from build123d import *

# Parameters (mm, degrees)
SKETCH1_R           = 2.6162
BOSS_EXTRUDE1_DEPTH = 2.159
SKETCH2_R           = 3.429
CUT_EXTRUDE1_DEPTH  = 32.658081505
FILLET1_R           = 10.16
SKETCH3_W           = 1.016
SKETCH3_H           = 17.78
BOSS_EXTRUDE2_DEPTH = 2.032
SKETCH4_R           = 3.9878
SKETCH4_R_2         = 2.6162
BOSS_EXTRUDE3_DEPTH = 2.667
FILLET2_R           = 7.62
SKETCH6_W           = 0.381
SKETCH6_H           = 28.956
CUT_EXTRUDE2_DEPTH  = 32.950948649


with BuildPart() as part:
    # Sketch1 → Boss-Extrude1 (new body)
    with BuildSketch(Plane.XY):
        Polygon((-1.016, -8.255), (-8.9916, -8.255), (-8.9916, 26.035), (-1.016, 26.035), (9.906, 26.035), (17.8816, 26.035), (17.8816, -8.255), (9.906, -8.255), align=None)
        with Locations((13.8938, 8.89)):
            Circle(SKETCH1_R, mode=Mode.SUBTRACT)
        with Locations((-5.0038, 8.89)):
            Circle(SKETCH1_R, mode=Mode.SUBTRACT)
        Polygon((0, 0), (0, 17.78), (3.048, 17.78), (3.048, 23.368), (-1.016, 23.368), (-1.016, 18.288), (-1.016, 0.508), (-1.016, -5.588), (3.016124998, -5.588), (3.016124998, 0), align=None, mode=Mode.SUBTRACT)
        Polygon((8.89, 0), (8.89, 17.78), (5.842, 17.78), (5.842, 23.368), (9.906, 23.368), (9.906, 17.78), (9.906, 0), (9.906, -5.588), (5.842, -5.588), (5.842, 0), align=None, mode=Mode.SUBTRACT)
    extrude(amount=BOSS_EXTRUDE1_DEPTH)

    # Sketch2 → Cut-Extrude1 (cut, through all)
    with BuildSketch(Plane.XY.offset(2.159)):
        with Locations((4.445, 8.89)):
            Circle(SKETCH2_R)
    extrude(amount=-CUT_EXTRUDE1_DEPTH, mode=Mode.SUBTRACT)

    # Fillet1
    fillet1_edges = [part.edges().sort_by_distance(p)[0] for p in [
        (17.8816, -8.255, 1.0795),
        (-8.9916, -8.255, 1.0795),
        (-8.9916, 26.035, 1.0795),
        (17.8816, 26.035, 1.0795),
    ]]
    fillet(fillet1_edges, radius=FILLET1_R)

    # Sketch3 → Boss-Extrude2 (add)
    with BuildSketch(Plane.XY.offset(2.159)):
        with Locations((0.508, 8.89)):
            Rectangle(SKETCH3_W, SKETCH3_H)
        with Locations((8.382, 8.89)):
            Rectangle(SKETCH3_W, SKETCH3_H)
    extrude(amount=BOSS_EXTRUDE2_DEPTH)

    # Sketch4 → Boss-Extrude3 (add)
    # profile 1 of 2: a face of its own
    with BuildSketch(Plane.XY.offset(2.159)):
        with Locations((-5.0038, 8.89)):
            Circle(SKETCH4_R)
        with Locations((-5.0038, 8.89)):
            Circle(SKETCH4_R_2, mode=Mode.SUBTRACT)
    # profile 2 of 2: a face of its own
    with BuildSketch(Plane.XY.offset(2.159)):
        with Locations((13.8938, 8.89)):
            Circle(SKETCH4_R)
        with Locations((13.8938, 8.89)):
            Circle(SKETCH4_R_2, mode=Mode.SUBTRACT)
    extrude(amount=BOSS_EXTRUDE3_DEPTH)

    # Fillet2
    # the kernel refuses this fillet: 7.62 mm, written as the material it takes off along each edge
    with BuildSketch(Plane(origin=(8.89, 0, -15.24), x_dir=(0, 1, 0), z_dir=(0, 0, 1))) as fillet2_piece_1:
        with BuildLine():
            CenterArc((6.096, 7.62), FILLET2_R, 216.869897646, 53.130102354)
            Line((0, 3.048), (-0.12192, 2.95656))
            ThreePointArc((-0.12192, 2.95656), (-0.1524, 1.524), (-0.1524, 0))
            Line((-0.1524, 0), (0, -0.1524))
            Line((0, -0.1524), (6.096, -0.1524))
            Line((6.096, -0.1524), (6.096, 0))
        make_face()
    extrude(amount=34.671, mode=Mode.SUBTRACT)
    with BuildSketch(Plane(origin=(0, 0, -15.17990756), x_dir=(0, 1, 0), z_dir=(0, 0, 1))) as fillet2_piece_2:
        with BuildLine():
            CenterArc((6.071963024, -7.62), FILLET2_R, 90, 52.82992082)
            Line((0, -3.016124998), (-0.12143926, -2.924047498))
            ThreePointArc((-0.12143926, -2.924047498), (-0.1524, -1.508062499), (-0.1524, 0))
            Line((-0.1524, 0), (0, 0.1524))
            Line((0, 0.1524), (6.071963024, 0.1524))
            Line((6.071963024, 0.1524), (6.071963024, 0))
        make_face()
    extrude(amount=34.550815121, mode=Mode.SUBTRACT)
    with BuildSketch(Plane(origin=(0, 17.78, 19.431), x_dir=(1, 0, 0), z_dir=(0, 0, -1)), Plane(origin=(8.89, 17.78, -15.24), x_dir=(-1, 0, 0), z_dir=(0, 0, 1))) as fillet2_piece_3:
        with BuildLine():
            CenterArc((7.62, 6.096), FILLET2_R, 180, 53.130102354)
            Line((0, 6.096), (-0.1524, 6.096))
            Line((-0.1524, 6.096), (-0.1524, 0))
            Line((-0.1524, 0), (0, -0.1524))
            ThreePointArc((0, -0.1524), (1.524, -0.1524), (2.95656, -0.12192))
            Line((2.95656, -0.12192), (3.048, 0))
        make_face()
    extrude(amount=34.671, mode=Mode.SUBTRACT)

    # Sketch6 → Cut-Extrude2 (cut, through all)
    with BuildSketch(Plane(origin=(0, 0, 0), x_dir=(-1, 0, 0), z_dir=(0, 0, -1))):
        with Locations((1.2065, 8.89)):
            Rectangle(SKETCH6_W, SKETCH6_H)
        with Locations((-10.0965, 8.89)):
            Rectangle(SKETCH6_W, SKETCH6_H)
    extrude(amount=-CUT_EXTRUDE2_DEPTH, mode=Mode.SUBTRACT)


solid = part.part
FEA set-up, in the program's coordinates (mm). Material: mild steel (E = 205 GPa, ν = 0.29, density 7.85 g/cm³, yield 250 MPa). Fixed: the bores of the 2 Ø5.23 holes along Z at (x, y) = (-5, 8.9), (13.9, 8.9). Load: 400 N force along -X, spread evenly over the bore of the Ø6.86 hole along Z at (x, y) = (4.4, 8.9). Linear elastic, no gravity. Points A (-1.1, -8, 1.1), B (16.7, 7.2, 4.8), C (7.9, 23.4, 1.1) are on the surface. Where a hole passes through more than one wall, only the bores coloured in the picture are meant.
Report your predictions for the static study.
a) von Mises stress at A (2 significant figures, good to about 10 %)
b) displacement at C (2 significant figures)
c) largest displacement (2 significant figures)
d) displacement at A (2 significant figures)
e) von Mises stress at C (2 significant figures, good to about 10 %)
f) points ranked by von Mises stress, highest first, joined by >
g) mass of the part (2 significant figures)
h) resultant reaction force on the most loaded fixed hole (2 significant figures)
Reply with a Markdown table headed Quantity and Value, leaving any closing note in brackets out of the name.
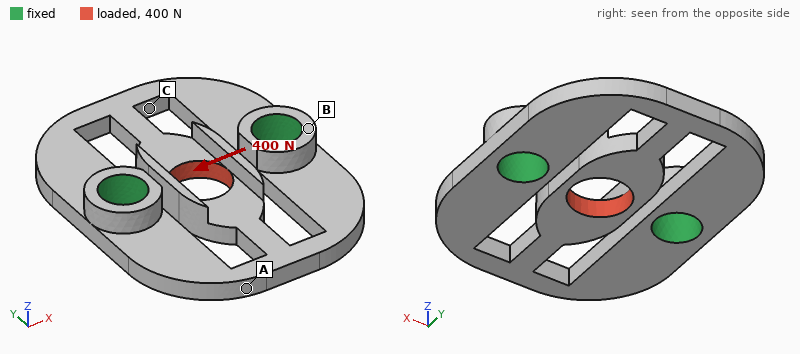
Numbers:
| Quantity | Value |
|---|---|
| von Mises stress at A | 51 MPa |
| displacement at C | 8.9 µm |
| largest displacement | 30 µm |
| displacement at A | 8.7 µm |
| von Mises stress at C | 110 MPa |
| points ranked by von Mises stress, highest first, joined by > | C > A > B |
| mass of the part | 11 g |
| resultant reaction force on the most loaded fixed hole | 200 N |
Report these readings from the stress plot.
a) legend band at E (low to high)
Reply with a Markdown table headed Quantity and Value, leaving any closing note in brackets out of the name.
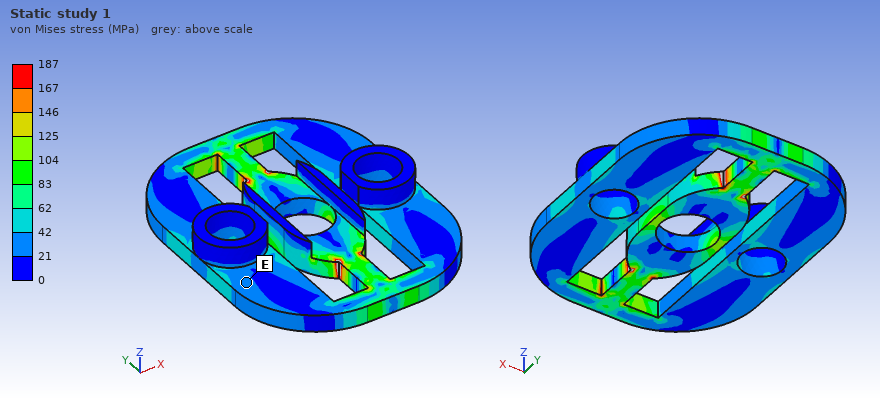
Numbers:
| Quantity | Value |
|---|---|
| legend band at E | 21 to 42 MPa |
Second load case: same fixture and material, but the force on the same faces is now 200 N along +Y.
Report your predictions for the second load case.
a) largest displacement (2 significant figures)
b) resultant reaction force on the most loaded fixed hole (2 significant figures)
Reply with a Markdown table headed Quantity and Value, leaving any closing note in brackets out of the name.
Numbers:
| Quantity | Value |
|---|---|
| largest displacement | 4.3 µm |
| resultant reaction force on the most loaded fixed hole | 100 N |
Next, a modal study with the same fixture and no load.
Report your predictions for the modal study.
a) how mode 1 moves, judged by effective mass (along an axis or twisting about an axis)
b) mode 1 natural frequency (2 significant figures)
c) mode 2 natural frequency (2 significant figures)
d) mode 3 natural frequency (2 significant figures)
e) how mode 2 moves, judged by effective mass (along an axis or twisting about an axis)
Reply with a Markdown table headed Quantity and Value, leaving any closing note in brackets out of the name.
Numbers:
| Quantity | Value |
|---|---|
| how mode 1 moves, judged by effective mass | along Z |
| mode 1 natural frequency | 5500 Hz |
| mode 2 natural frequency | 7600 Hz |
| mode 3 natural frequency | 10 kHz |
| how mode 2 moves, judged by effective mass | twisting about X |
